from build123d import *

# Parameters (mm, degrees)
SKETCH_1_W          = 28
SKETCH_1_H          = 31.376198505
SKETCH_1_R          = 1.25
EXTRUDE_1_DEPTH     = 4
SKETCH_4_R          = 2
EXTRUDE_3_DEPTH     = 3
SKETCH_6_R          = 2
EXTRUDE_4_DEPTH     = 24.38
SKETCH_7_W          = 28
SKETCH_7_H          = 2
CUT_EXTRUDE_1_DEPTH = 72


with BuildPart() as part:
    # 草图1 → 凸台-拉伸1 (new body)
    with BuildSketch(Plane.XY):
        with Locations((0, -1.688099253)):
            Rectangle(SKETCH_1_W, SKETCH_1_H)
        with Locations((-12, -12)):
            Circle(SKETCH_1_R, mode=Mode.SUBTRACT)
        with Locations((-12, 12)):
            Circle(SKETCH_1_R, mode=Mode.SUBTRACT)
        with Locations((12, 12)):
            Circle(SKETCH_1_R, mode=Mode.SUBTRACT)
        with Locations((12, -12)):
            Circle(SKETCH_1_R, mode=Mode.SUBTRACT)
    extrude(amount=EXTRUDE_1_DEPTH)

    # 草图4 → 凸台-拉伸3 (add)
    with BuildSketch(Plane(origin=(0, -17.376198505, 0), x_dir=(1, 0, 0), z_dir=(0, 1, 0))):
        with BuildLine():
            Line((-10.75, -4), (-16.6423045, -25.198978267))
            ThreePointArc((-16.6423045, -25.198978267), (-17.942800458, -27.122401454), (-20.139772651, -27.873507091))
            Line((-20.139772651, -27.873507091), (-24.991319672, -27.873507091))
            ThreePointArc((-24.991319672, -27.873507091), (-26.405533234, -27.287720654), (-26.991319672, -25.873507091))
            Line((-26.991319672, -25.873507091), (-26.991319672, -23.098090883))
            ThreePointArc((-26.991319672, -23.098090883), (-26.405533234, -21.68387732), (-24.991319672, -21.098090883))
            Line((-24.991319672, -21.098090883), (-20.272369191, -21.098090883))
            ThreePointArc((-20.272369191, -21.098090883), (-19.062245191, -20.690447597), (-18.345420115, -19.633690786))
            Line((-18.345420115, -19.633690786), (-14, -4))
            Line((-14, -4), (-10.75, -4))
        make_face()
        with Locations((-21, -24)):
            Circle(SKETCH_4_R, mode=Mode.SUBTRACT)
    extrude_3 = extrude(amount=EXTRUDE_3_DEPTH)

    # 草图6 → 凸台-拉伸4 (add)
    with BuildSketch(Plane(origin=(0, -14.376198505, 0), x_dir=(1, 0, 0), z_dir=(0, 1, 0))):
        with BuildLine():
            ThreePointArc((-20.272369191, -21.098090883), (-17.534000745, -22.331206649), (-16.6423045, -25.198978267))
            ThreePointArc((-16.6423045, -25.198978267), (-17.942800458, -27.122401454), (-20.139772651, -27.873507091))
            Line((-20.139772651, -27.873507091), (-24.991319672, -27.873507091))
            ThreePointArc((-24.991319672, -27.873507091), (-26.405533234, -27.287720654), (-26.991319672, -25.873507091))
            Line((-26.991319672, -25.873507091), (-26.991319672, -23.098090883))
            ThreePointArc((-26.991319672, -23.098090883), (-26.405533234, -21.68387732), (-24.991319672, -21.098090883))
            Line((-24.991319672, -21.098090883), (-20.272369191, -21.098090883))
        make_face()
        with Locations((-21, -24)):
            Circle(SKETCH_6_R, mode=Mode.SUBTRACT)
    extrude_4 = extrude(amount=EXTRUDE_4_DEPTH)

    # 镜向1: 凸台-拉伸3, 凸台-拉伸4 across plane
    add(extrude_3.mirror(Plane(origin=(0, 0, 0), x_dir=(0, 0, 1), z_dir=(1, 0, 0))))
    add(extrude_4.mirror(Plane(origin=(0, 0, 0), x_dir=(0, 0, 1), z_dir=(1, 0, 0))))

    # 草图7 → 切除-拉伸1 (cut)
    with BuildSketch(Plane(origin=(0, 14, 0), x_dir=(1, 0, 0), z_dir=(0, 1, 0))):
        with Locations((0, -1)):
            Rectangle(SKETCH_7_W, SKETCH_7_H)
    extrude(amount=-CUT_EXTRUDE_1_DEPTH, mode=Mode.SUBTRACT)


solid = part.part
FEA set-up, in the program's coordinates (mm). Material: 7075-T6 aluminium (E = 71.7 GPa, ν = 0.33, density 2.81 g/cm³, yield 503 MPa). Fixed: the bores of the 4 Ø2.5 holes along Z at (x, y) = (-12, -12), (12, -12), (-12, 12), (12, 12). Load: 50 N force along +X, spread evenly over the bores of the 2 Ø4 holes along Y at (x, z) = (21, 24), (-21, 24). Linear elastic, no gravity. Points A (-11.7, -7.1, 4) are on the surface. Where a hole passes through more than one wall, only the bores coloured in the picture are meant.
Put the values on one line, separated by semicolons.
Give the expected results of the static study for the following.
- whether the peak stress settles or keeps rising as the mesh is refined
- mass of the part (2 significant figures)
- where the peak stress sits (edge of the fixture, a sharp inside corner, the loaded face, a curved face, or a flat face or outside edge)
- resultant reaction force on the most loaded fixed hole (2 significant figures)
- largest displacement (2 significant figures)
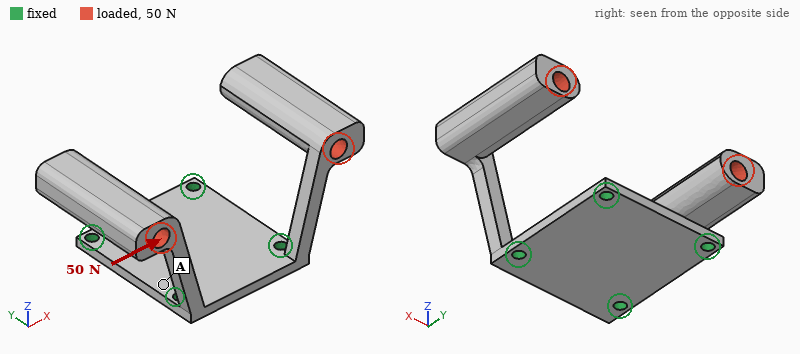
keeps rising; 14 g; edge of the fixture; 35 N; 0.75 mm
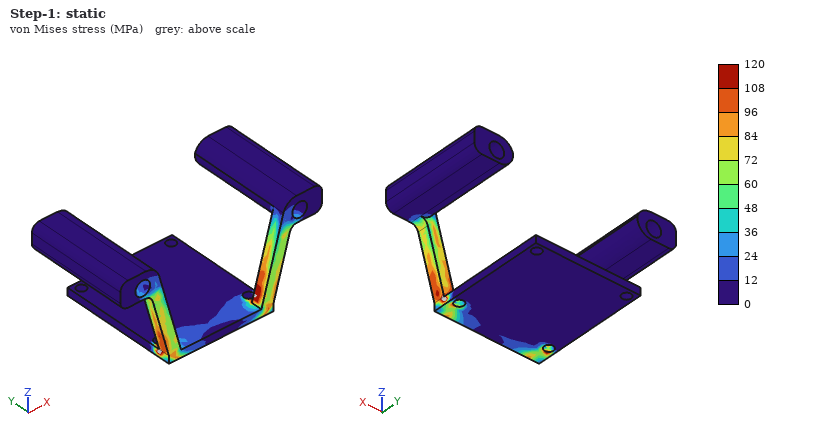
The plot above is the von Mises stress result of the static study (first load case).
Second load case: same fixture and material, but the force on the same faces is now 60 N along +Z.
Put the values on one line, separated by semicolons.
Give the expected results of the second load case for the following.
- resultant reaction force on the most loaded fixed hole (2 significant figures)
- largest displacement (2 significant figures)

27 N; 0.64 mm
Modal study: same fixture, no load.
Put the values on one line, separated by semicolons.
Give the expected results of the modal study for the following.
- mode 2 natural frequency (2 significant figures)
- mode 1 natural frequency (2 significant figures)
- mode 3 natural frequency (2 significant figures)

530 Hz; 520 Hz; 550 Hz
